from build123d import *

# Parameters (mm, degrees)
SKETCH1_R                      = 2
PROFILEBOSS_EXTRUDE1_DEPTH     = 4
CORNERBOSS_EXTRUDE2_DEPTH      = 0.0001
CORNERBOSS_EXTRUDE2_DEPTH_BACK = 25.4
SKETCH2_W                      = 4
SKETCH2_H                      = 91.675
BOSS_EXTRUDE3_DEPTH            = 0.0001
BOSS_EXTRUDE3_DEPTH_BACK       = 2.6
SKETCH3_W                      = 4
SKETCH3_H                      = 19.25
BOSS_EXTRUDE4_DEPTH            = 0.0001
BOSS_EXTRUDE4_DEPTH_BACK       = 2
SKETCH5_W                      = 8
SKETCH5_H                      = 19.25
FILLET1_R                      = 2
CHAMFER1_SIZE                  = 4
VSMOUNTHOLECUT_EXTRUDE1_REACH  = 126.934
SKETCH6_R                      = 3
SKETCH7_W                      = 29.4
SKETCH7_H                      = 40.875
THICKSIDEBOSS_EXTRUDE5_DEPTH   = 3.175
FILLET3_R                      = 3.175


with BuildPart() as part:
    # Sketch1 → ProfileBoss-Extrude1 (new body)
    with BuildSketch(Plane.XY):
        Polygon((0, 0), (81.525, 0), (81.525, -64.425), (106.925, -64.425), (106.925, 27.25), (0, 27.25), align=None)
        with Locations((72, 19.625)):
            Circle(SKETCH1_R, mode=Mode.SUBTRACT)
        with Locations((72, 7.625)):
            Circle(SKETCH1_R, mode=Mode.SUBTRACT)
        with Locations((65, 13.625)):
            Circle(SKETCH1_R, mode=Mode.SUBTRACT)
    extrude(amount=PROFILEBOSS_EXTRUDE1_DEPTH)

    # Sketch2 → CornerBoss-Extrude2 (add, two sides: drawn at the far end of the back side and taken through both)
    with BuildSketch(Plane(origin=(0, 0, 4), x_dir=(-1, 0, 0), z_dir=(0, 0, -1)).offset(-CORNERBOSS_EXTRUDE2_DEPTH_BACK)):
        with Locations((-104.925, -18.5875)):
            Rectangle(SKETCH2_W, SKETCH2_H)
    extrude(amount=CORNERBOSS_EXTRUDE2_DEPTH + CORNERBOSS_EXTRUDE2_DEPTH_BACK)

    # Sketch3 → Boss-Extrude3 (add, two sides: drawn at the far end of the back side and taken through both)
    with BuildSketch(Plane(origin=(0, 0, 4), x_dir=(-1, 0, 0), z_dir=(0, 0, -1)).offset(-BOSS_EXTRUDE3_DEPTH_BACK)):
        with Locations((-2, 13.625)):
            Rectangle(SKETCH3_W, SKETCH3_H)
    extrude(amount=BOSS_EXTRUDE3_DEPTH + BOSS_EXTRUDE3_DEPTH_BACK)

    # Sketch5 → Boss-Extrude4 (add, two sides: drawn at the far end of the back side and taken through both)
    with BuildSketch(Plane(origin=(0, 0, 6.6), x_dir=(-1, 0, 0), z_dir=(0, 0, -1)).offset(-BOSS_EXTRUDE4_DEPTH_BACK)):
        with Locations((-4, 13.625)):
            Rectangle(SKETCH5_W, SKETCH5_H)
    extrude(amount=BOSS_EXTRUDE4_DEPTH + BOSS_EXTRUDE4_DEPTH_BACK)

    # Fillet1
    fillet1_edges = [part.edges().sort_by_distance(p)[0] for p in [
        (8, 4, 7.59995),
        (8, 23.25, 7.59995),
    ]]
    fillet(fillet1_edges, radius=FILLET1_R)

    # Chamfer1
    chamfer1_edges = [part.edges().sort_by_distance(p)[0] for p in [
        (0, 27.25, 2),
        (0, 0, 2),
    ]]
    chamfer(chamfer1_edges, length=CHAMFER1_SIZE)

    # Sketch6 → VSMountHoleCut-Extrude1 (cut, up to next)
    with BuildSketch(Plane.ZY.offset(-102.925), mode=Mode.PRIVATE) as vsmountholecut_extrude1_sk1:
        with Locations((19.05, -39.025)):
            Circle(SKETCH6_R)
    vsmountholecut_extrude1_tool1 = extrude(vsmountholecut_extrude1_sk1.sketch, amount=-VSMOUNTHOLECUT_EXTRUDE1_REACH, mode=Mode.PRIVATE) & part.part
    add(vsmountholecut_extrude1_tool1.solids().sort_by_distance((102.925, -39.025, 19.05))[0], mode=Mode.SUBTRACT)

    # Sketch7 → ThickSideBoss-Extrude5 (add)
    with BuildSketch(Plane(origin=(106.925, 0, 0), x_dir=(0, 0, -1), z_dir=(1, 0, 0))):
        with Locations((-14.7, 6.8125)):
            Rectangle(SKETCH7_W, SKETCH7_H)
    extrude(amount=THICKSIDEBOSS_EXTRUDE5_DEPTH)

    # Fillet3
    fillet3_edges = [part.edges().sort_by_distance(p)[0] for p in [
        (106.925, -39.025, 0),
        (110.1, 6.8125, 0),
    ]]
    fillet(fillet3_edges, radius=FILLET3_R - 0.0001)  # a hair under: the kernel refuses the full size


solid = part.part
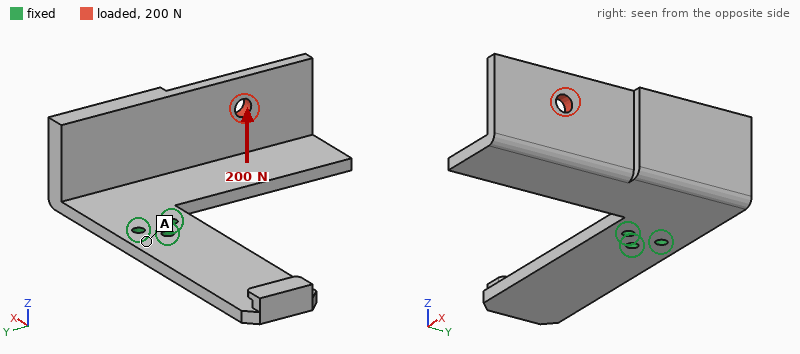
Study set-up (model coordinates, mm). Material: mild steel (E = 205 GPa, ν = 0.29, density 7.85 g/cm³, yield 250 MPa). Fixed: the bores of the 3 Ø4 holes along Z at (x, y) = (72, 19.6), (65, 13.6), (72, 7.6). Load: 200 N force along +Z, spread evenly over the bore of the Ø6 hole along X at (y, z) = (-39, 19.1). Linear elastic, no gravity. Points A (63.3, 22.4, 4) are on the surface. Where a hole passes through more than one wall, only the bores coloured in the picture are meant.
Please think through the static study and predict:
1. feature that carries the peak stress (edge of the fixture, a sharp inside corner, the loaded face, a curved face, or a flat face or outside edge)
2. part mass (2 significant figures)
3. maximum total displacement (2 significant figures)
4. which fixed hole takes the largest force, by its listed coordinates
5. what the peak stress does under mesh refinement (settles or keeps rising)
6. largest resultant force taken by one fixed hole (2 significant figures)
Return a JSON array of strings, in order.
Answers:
["edge of the fixture", "250 g", "0.44 mm", "(72, 7.6)", "keeps rising", "760 N"]
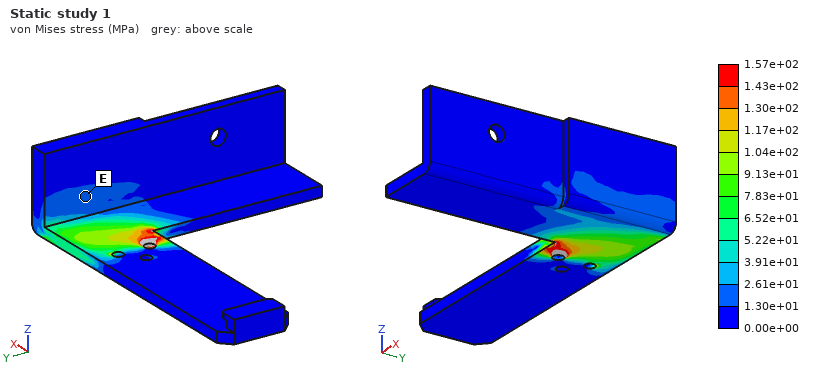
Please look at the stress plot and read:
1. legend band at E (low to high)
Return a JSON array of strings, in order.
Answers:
["1.30e+01 to 2.61e+01 MPa"]
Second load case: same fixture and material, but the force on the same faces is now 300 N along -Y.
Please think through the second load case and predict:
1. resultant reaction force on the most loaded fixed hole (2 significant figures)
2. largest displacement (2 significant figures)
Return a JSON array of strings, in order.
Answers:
["680 N", "0.17 mm"]
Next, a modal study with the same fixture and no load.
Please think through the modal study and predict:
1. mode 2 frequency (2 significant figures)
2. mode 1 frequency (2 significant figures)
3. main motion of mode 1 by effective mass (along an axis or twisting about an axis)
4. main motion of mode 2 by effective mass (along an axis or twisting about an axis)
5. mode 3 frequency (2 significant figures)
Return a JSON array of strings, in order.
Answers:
["710 Hz", "430 Hz", "along Z", "along Z", "810 Hz"]
